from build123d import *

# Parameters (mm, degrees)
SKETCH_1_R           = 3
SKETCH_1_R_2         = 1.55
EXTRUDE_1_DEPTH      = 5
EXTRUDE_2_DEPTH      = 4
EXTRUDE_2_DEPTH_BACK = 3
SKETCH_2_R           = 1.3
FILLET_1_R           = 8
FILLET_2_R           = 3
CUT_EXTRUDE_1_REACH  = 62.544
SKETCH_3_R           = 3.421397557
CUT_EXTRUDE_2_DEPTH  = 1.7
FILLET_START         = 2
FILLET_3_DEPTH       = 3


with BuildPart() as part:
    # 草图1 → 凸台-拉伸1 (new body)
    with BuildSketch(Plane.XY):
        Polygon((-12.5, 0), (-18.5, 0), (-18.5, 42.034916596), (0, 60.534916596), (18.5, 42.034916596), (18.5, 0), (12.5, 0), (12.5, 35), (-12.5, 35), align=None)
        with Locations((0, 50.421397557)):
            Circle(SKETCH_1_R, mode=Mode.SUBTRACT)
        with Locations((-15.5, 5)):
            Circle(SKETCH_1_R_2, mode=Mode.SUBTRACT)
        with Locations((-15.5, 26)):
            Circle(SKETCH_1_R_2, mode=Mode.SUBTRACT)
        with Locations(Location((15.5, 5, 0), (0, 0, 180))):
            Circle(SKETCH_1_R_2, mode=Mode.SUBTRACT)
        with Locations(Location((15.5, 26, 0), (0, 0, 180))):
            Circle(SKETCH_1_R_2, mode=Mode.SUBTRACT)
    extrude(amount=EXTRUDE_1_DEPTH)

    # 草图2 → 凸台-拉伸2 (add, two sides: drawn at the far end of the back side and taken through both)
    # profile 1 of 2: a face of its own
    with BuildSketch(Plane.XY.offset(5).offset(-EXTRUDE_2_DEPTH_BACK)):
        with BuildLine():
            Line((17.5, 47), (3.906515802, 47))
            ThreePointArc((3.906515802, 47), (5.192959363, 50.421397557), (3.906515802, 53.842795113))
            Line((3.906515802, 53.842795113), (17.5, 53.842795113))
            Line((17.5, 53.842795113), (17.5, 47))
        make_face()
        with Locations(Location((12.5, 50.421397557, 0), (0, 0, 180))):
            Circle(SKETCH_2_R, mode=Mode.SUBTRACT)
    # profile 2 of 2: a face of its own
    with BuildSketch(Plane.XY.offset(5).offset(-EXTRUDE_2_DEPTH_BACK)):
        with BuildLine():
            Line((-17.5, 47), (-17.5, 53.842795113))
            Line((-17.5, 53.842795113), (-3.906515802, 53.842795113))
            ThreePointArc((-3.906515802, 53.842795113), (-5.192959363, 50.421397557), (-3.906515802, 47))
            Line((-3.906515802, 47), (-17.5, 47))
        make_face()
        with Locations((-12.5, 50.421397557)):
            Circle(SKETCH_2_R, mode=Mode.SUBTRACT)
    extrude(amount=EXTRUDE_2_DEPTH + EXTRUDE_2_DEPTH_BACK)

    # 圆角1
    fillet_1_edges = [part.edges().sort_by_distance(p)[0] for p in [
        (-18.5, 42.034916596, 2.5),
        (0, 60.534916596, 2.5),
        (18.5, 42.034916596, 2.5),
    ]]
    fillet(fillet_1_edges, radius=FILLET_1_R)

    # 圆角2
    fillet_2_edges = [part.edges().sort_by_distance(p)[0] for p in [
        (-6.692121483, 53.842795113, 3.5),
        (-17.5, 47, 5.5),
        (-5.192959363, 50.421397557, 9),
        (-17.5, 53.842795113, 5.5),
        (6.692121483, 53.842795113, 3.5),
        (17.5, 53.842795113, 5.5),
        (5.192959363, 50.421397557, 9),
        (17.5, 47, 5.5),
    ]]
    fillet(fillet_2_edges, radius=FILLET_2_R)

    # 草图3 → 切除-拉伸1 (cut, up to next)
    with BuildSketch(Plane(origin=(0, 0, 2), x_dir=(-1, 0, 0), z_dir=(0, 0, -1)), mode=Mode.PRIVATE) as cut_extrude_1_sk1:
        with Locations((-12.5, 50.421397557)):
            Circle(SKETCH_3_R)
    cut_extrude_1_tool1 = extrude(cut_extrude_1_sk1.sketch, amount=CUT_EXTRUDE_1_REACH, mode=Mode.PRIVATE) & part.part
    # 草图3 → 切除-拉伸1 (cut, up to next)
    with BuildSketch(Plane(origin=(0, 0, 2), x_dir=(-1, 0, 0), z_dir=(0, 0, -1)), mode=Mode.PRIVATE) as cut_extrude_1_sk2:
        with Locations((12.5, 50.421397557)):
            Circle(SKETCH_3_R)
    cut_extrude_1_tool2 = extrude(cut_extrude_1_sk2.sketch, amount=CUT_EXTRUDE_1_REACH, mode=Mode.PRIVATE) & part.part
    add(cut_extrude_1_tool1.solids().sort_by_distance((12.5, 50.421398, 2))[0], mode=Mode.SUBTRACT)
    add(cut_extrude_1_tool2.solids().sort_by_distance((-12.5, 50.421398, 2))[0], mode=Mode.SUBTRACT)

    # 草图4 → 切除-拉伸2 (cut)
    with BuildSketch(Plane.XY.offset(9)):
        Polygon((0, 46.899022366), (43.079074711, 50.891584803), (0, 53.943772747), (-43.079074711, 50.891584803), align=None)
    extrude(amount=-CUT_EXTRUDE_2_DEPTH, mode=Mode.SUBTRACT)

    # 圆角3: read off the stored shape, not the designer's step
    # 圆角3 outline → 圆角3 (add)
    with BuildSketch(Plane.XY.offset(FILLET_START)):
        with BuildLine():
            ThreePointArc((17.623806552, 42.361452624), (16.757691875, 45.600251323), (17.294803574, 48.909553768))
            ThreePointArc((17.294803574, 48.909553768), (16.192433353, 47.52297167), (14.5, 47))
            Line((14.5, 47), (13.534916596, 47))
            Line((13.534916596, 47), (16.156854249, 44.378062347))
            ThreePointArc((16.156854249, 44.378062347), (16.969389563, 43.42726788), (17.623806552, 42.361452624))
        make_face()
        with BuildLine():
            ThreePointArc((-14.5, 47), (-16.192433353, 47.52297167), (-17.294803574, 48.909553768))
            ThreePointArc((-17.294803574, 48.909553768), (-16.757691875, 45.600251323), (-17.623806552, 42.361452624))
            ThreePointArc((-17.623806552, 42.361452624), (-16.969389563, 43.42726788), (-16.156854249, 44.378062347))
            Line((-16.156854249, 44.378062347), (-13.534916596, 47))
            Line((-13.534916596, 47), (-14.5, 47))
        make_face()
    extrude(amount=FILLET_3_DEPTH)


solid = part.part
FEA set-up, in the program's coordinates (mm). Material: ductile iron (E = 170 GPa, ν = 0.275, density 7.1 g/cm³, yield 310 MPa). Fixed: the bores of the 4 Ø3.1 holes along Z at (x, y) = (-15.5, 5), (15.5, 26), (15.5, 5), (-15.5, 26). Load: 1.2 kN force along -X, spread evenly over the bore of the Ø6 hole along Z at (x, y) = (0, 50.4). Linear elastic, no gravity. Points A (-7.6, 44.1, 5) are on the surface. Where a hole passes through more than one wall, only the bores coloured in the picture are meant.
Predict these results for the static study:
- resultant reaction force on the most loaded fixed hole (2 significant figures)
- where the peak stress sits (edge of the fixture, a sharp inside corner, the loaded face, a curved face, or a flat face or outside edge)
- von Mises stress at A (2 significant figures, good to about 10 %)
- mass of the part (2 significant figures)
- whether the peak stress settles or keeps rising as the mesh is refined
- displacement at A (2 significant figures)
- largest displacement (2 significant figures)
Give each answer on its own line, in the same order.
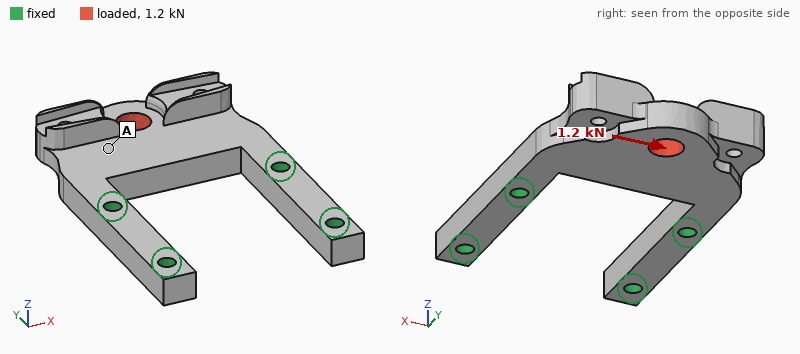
940 N
edge of the fixture
16 MPa
38 g
keeps rising
11 µm
14 µm
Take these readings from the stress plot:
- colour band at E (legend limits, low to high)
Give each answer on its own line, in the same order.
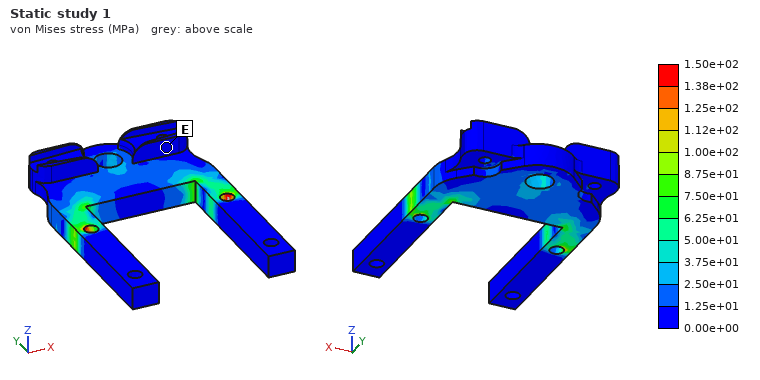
0.00e+00 to 1.25e+01 MPa
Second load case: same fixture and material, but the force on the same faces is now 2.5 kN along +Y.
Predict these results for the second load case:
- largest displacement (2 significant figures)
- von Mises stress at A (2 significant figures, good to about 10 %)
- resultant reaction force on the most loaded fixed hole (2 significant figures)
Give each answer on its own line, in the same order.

9.2 µm
26 MPa
1.3 kN
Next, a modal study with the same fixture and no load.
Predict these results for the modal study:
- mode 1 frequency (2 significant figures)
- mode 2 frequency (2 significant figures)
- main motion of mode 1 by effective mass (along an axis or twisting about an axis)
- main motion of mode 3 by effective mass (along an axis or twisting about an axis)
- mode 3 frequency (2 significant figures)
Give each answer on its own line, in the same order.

2900 Hz
9000 Hz
along Z
along X
11 kHz
